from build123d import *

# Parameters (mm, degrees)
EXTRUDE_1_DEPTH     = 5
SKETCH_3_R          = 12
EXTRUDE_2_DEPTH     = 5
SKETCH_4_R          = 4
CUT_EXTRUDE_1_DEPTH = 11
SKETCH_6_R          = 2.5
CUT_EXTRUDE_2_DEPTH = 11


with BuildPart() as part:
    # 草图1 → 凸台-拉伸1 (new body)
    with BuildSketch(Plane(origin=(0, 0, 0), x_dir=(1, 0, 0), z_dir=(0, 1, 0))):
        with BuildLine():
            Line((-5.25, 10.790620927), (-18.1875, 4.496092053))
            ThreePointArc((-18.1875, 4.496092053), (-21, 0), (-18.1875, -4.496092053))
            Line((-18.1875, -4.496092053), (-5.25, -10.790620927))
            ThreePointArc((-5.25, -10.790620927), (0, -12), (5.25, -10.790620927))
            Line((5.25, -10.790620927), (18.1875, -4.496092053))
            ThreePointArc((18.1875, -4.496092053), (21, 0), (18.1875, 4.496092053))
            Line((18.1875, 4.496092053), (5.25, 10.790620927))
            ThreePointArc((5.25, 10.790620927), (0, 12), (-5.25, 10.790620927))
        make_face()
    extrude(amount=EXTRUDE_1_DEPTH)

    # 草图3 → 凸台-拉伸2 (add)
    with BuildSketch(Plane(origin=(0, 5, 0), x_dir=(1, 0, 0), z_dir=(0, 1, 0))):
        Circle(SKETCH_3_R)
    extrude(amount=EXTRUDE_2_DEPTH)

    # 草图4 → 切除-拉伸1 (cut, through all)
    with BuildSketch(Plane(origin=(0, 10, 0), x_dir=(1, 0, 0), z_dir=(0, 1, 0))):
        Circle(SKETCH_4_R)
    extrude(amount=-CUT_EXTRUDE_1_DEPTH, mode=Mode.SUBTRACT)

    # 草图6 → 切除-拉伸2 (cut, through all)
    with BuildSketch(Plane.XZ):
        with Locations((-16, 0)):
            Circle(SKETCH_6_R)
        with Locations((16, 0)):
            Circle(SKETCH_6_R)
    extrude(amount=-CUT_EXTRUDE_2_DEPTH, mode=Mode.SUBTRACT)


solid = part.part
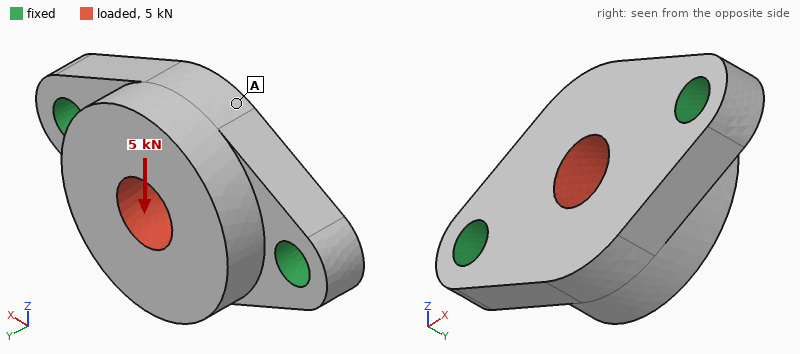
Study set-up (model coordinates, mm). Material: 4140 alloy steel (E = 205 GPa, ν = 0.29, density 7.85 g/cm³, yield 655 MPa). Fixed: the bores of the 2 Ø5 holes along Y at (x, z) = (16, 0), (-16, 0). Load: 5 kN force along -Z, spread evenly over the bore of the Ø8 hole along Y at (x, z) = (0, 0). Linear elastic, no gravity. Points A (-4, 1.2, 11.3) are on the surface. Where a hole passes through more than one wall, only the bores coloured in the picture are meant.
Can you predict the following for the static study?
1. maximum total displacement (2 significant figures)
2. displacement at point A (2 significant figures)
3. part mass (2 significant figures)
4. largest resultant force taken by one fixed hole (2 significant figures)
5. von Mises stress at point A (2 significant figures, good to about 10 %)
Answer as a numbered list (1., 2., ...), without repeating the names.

1. 14 µm
2. 8.8 µm
3. 39 g
4. 2.5 kN
5. 33 MPa
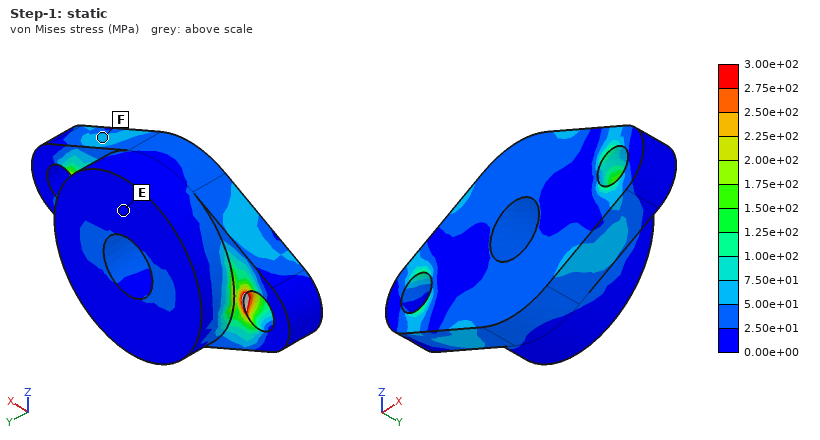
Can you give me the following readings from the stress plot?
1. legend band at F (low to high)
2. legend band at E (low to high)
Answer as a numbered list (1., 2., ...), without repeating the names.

1. 5.00e+01 to 7.50e+01 MPa
2. 0.00e+00 to 2.50e+01 MPa
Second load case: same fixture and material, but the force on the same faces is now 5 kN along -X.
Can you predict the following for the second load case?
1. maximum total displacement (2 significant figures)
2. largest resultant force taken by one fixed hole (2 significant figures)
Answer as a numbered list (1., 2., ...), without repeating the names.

1. 2.5 µm
2. 2.5 kN
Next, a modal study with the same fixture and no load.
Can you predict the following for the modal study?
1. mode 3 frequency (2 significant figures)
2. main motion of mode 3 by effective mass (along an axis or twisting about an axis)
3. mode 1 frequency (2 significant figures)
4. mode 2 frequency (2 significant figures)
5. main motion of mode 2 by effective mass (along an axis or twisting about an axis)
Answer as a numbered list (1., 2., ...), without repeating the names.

1. 34 kHz
2. along Z
3. 15 kHz
4. 23 kHz
5. along Y
